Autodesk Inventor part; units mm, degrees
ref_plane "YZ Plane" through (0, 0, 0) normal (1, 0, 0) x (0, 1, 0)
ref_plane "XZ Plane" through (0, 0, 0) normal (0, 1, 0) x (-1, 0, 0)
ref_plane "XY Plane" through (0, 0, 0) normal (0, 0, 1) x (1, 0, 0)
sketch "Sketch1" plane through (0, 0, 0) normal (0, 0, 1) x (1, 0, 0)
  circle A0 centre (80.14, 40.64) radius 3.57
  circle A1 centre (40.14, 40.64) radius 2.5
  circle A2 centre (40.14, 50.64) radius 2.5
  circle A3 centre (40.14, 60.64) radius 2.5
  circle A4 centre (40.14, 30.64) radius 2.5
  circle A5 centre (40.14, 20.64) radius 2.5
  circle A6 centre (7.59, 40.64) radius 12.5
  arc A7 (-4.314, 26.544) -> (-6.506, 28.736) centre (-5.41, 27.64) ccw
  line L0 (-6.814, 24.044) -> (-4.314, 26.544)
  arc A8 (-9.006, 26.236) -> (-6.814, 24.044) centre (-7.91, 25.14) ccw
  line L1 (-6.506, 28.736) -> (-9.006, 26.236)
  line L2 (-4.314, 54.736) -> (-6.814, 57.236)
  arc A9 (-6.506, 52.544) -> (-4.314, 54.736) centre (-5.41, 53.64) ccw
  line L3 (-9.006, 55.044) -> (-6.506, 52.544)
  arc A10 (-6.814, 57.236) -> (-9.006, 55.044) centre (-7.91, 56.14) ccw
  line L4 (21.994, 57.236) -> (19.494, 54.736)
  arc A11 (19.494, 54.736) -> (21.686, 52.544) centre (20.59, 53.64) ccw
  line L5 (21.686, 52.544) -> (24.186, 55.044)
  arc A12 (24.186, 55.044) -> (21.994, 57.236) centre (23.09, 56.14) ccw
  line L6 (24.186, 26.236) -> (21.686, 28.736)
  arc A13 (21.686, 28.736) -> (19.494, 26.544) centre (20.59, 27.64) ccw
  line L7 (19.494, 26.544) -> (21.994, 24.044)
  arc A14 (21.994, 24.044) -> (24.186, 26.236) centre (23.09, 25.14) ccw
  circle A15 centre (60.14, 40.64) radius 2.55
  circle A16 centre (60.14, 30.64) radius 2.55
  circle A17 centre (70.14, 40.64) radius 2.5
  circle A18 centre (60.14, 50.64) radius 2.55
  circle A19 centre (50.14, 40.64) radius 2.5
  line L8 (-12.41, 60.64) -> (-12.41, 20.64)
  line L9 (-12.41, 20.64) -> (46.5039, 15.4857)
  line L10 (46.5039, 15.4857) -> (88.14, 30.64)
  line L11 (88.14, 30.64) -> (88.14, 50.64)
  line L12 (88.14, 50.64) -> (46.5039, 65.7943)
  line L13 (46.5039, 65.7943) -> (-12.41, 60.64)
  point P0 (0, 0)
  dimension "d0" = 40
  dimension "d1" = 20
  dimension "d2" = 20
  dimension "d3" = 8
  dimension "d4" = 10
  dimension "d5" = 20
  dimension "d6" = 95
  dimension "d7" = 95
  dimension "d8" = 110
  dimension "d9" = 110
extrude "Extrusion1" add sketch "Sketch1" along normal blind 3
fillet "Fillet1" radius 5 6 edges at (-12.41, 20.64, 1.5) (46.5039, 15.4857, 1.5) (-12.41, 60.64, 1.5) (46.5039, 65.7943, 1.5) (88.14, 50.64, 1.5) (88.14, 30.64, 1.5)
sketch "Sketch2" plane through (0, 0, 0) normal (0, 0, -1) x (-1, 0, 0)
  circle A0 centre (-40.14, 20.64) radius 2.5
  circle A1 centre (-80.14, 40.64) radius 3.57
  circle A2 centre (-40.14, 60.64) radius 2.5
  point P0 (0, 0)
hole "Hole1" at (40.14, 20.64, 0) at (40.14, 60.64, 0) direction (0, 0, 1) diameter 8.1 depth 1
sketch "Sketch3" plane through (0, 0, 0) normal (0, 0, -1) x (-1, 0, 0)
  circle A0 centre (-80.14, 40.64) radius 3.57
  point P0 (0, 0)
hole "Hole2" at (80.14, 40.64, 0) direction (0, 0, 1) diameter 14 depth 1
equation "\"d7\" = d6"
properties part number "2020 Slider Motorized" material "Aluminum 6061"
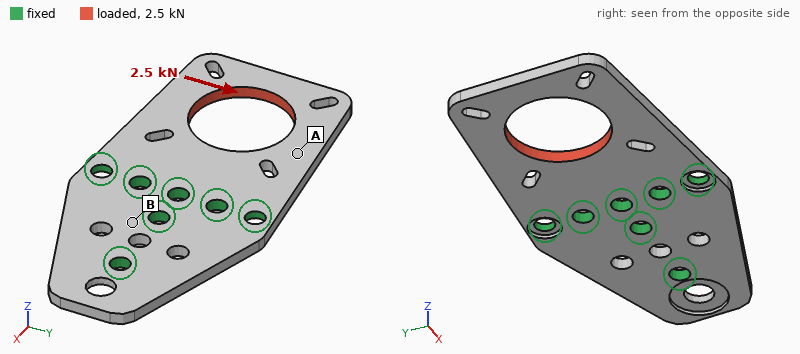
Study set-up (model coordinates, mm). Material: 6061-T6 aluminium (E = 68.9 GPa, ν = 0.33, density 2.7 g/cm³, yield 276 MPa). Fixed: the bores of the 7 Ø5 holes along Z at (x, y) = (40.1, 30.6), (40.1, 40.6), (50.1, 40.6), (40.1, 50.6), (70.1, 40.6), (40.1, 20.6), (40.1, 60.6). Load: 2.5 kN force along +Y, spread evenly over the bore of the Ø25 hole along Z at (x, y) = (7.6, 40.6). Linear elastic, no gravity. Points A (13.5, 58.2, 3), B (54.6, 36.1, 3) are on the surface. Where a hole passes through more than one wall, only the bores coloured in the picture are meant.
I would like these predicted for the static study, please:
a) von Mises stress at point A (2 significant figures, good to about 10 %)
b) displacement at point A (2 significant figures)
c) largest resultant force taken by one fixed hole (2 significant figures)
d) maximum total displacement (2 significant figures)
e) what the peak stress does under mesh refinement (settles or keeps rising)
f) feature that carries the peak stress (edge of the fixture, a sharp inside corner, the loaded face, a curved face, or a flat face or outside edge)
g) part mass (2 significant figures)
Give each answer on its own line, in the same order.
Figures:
51 MPa
0.050 mm
1.6 kN
0.13 mm
keeps rising
edge of the fixture
26 g
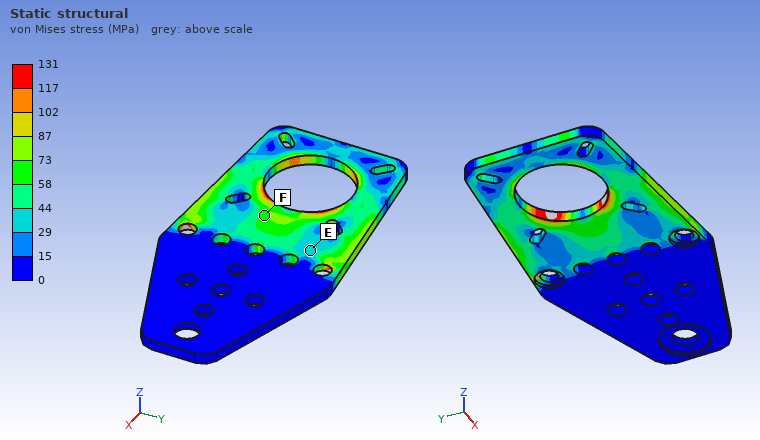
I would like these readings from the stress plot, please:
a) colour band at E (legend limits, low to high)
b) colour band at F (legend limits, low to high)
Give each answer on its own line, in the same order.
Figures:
29 to 44 MPa
58 to 73 MPa
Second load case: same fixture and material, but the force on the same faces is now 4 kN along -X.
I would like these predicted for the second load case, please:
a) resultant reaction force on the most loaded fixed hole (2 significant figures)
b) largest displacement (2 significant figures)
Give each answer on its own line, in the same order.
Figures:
1.0 kN
54 µm
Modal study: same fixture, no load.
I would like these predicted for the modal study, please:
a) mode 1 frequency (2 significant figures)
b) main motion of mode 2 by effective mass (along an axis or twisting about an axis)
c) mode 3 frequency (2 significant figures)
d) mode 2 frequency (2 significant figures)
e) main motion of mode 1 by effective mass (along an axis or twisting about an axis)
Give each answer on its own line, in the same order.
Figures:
1000 Hz
twisting about X
5300 Hz
2400 Hz
along Z
